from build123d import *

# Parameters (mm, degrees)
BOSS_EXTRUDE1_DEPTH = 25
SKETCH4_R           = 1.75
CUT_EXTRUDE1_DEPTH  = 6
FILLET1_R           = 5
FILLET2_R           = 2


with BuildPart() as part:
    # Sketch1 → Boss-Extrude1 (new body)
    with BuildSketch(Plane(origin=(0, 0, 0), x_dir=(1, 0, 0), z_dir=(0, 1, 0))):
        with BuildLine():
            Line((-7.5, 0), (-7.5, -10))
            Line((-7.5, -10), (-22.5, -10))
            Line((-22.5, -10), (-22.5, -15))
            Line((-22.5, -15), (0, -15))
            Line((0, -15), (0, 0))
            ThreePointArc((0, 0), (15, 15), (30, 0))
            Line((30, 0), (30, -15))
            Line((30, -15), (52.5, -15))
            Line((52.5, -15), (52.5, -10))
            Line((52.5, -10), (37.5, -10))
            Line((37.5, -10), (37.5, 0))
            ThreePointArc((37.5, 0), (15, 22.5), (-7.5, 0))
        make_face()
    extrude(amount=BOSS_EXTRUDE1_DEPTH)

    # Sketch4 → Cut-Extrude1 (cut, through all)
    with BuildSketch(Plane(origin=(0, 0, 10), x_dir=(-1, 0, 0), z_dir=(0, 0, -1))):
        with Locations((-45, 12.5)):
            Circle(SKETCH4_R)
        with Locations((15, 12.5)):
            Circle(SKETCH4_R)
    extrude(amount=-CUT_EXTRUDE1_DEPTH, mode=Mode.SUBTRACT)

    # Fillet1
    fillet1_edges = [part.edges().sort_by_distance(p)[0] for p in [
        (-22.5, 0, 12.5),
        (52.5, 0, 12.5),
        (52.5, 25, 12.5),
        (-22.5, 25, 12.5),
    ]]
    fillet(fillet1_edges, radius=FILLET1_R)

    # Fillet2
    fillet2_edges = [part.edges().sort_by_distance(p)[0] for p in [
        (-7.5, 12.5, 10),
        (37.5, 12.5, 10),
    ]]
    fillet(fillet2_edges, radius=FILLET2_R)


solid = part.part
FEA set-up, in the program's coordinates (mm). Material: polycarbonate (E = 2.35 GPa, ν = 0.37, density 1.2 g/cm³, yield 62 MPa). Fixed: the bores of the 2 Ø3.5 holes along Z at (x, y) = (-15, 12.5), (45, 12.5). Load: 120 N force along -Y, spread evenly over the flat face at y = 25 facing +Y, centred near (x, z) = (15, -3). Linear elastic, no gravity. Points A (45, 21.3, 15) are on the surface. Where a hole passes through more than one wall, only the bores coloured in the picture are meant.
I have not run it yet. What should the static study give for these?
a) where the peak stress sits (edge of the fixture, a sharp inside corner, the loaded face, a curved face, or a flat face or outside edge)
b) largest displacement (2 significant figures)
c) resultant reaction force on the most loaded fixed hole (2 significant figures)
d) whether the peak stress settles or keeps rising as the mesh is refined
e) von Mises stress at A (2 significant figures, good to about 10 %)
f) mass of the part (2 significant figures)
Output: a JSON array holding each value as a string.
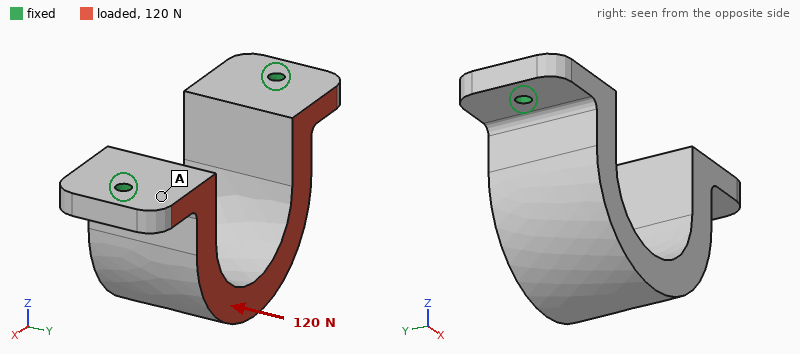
["edge of the fixture", "0.44 mm", "60 N", "keeps rising", "3.2 MPa", "24 g"]
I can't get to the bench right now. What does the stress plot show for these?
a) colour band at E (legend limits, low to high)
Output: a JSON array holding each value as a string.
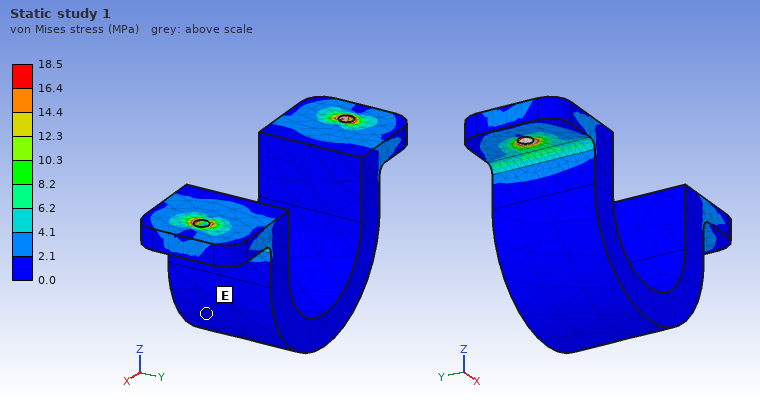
["0.0 to 2.1 MPa"]
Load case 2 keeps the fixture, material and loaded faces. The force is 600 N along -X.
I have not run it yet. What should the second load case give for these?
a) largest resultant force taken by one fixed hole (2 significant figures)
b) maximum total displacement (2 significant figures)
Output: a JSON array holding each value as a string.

["350 N", "0.49 mm"]
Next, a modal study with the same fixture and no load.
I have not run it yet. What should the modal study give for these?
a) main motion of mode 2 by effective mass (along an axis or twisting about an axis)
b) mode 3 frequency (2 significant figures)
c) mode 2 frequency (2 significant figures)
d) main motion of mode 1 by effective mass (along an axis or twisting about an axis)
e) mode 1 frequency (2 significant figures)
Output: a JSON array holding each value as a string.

["along X", "2400 Hz", "1700 Hz", "along Y", "640 Hz"]
